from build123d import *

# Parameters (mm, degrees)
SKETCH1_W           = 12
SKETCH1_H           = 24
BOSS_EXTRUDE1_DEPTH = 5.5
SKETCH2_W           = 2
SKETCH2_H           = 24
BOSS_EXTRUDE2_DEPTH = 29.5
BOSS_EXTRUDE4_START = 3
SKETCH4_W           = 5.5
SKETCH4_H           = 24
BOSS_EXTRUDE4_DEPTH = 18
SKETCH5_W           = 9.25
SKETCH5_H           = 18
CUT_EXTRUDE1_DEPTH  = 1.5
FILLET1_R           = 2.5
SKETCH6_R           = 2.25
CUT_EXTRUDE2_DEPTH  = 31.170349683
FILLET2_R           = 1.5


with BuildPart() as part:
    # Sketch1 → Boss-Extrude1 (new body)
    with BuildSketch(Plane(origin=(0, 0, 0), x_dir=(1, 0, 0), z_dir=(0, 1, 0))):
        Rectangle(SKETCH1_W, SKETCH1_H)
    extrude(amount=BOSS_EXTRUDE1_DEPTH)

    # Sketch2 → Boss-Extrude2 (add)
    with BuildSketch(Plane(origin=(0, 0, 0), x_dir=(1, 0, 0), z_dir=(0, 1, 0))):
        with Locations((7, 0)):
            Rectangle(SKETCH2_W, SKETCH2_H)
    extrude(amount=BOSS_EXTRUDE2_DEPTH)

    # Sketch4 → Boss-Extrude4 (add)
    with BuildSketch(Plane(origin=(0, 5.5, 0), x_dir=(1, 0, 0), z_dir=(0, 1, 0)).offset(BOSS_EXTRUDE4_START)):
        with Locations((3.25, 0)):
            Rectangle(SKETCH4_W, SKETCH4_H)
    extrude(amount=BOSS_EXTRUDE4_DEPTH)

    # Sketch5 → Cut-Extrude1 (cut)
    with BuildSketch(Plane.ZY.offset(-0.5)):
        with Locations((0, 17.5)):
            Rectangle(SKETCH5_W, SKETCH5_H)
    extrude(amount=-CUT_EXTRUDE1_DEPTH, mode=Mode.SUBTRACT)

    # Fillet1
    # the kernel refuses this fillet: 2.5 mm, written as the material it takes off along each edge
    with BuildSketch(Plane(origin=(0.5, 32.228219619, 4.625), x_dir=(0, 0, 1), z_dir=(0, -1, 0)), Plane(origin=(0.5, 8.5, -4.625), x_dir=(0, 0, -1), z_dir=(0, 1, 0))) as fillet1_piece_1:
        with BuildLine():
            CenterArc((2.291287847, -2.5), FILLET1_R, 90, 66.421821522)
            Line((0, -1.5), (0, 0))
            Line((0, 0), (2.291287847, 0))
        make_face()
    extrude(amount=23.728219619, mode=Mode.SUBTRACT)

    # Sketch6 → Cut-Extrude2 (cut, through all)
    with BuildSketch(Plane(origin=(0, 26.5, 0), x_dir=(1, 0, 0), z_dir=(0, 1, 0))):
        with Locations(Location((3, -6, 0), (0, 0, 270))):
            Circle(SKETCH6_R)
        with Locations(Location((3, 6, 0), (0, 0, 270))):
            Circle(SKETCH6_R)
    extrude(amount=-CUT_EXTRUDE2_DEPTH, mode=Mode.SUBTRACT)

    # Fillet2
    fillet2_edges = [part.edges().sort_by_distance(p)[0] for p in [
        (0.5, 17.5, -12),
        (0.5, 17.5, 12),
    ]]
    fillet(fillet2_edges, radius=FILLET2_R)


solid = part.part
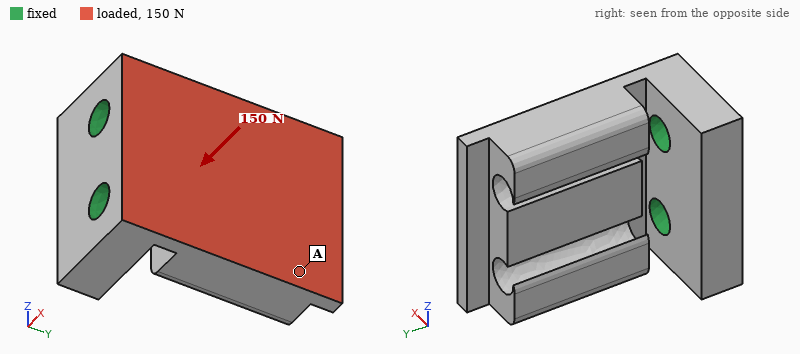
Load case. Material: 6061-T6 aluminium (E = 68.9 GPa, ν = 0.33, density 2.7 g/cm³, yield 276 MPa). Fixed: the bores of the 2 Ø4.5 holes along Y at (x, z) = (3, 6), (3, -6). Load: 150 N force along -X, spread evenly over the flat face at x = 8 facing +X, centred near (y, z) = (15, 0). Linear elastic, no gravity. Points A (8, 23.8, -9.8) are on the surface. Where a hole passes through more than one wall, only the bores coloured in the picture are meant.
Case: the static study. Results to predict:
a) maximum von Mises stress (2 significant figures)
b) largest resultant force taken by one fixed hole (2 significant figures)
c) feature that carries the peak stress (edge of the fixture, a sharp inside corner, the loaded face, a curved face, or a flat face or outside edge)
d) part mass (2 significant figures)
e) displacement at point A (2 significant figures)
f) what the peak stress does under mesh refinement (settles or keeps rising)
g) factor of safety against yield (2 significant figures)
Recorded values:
79 MPa
75 N
the loaded face
12 g
0.098 mm
settles
3.5
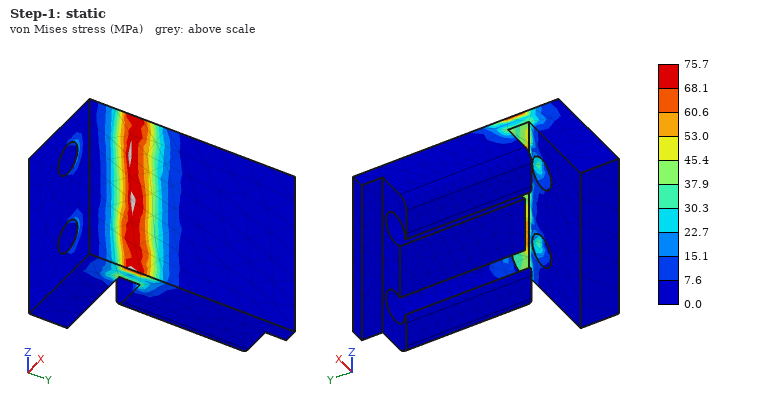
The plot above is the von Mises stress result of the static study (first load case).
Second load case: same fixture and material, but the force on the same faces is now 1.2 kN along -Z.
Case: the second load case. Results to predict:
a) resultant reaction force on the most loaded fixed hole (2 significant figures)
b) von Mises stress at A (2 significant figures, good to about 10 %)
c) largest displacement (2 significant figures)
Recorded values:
1.1 kN
11 MPa
44 µm
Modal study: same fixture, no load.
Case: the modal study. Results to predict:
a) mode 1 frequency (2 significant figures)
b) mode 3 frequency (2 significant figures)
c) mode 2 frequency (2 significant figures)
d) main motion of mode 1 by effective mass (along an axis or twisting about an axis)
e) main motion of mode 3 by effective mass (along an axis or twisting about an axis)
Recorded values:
2300 Hz
12 kHz
8600 Hz
along X
along Z
